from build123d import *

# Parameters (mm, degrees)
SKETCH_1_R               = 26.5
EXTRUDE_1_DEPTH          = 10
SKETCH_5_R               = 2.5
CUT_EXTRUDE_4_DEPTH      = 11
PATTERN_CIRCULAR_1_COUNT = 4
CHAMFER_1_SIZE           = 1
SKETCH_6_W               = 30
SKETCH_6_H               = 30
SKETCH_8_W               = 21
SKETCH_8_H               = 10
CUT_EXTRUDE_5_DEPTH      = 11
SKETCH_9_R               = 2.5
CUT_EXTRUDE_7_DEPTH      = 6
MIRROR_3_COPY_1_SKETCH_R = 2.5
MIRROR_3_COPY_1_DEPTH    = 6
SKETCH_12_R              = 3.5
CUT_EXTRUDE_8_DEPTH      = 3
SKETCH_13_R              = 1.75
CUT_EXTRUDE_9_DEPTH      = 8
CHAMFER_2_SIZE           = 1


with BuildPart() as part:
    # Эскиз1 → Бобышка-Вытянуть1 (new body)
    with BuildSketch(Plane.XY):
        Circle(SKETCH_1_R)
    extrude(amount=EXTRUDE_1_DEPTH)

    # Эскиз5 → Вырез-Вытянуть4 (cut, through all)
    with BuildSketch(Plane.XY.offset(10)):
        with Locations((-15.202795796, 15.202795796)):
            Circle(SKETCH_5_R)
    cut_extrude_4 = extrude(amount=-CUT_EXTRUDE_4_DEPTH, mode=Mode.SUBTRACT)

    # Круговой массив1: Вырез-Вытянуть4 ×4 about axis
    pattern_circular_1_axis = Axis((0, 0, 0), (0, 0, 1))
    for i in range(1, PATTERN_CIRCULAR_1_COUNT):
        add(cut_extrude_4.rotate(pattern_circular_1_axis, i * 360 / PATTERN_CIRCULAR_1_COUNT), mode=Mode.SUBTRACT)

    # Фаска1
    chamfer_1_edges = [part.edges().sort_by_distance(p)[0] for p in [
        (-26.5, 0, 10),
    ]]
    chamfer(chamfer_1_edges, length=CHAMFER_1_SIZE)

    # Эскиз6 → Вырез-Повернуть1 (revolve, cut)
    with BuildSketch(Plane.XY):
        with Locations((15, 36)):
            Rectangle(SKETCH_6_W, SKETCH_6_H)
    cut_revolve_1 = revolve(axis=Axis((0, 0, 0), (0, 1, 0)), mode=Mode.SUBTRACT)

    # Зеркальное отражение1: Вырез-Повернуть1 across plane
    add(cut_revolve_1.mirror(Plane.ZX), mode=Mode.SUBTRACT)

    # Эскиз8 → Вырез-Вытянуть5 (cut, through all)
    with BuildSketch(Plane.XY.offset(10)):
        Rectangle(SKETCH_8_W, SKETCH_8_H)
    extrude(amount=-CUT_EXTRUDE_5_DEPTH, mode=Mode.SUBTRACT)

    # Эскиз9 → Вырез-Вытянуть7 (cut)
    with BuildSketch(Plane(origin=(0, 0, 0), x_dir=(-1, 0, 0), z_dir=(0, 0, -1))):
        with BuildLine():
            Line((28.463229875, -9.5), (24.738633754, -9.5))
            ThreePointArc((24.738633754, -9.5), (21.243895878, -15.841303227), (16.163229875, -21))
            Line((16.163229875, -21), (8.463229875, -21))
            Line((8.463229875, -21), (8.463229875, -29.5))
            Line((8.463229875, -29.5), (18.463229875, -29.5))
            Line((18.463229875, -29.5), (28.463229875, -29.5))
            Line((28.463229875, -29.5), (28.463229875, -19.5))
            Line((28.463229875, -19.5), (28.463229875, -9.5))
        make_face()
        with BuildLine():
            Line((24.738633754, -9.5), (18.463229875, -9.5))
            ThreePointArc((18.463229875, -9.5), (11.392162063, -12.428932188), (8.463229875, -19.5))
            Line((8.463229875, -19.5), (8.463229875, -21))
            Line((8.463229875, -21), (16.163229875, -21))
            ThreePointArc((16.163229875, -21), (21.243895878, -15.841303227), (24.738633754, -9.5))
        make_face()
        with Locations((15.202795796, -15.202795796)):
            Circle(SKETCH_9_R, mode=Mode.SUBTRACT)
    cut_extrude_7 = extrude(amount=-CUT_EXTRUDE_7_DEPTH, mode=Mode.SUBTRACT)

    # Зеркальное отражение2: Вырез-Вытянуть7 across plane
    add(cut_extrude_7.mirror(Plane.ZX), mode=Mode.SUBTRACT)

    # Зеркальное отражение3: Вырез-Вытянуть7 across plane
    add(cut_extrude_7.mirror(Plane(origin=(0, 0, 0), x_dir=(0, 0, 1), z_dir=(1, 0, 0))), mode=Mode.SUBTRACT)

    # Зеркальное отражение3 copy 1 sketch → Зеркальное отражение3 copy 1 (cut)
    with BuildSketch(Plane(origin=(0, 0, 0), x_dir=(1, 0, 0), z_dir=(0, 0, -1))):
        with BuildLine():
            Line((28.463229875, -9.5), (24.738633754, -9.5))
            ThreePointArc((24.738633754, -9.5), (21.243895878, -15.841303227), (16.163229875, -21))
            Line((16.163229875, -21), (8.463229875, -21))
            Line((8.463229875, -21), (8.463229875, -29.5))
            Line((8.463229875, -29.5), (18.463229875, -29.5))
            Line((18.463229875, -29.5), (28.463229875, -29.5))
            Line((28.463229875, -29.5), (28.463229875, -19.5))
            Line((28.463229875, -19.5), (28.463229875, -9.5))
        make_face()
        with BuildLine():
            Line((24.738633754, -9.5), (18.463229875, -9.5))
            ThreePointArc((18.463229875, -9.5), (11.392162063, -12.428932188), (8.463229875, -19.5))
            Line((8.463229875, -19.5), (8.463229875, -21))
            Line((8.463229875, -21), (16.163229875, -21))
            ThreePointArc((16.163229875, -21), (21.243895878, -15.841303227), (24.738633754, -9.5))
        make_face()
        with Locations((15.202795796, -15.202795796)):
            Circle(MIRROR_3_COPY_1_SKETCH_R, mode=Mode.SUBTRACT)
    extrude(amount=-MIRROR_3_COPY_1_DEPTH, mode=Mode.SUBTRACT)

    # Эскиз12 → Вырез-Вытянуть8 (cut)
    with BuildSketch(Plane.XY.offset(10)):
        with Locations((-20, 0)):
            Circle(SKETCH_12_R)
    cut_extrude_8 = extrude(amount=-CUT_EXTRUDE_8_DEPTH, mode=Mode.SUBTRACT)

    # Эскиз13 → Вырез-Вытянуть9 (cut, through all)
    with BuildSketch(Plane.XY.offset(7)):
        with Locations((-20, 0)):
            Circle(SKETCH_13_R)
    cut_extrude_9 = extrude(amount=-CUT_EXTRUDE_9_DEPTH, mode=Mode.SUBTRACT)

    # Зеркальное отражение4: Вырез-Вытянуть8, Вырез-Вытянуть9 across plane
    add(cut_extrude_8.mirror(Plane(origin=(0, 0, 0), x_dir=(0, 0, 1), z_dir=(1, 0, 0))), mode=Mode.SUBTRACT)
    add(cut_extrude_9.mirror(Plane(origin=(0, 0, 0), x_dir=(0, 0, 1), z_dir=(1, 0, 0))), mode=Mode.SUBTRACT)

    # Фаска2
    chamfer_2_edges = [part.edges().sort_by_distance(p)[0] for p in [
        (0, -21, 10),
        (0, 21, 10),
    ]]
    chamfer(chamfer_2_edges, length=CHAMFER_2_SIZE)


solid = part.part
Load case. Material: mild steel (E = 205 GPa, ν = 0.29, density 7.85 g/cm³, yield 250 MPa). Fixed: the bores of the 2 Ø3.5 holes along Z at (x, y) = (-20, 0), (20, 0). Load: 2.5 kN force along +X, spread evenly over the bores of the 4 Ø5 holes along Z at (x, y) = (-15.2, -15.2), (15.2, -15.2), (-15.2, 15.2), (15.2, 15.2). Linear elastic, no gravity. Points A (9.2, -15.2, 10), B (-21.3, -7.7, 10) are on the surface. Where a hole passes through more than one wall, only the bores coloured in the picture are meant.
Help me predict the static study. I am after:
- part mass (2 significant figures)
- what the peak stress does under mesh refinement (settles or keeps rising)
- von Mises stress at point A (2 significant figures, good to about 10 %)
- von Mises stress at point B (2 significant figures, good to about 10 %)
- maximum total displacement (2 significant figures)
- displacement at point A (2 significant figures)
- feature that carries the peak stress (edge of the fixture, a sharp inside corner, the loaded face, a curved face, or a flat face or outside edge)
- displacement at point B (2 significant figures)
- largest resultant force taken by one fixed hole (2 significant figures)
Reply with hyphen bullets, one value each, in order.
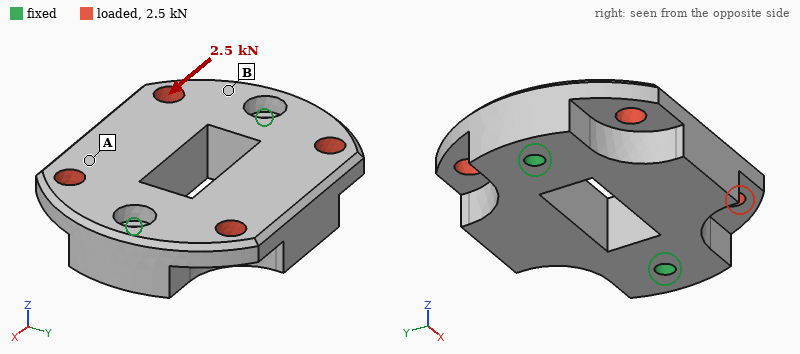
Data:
- 110 g
- keeps rising
- 11 MPa
- 4.3 MPa
- 2.0 µm
- 1.3 µm
- edge of the fixture
- 0.78 µm
- 1.3 kN
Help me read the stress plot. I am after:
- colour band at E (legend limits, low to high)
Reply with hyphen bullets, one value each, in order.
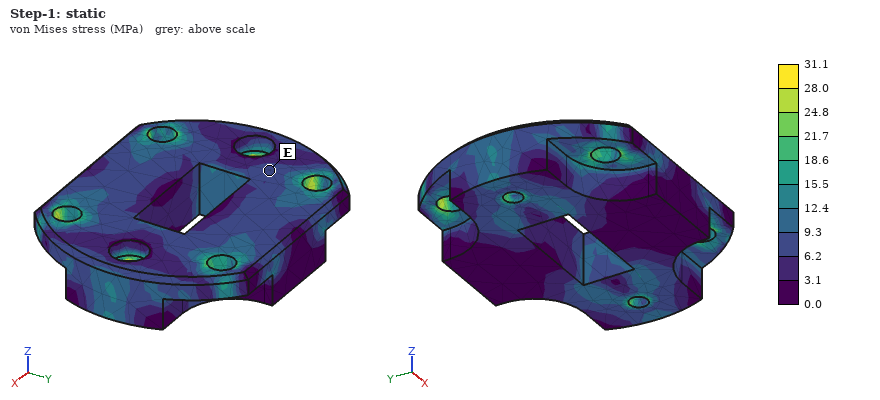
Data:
- 6.2 to 9.3 MPa
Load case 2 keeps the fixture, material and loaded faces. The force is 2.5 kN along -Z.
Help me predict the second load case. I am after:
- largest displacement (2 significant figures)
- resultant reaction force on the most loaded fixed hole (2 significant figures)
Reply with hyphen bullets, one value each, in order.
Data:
- 12 µm
- 1.3 kN
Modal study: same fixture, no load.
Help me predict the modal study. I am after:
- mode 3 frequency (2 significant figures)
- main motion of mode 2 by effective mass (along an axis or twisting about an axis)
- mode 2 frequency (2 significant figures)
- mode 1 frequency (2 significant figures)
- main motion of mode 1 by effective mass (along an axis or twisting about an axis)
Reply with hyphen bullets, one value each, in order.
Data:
- 22 kHz
- along Z
- 11 kHz
- 8400 Hz
- twisting about X
